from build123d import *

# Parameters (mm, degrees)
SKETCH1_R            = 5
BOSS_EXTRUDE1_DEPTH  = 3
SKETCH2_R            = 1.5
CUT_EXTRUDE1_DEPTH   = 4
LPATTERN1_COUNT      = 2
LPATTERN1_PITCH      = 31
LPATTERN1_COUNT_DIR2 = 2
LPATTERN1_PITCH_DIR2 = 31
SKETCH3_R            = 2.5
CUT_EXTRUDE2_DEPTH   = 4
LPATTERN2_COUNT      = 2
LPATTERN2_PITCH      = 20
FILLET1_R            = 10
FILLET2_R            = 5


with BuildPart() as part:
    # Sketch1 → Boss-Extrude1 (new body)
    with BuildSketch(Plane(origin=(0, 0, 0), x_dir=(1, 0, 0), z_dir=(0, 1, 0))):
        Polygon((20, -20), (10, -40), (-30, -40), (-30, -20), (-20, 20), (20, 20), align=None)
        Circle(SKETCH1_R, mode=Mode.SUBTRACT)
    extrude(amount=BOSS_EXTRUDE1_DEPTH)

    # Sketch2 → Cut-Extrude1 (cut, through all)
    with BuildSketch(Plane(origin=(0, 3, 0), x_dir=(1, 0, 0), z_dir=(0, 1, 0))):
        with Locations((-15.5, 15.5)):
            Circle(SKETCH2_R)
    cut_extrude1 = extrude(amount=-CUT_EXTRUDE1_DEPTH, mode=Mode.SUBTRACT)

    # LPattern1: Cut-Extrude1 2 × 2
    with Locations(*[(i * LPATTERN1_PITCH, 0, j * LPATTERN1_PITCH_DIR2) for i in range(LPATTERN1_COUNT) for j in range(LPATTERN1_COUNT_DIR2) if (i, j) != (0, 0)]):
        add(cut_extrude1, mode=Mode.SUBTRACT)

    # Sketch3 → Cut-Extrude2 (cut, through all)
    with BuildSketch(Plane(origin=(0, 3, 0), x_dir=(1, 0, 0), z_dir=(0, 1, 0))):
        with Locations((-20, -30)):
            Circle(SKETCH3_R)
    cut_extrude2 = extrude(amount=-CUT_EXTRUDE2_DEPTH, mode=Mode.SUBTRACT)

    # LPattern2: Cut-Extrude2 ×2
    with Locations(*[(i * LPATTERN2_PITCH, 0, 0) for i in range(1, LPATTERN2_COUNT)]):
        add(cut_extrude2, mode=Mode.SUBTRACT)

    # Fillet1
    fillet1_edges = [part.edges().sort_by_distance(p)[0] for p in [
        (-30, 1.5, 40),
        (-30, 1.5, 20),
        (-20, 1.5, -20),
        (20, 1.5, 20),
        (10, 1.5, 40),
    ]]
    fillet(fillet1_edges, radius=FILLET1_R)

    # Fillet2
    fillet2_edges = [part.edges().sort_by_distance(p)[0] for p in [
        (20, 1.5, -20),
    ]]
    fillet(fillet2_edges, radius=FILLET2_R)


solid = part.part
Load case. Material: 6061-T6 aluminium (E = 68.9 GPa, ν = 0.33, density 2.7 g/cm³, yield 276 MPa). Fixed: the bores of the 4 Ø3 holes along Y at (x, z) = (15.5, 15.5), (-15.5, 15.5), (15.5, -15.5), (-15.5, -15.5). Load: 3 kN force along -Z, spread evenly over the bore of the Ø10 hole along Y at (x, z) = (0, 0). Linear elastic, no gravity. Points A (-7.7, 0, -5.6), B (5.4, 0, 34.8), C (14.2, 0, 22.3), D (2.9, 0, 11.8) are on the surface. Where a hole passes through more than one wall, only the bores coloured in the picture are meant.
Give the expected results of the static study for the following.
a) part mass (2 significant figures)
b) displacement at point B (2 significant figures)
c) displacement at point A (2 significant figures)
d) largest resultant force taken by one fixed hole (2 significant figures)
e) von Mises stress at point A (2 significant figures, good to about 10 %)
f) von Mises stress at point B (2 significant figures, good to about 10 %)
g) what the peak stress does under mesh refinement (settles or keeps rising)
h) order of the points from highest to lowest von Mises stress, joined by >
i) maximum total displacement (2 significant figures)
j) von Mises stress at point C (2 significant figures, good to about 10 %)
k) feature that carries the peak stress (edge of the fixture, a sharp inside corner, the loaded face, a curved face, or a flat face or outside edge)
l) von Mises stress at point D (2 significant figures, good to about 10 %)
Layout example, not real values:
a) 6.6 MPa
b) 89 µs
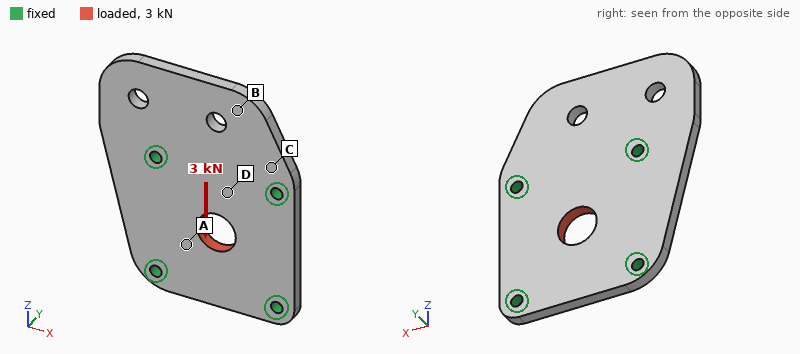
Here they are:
a) 20 g
b) 2.6 µm
c) 5.4 µm
d) 870 N
e) 24 MPa
f) 5.2 MPa
g) keeps rising
h) A > D > C > B
i) 9.7 µm
j) 11 MPa
k) edge of the fixture
l) 18 MPa
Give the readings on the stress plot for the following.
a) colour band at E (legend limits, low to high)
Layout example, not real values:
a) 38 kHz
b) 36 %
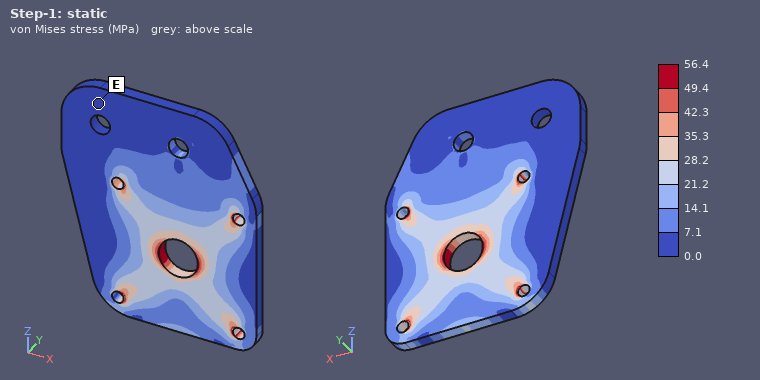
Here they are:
a) 0.0 to 7.1 MPa
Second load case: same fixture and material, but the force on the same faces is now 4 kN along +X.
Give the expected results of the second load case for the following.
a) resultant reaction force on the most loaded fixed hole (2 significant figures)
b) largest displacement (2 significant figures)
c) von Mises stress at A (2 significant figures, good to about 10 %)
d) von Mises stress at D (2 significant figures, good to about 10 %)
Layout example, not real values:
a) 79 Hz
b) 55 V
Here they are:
a) 1.2 kN
b) 13 µm
c) 33 MPa
d) 23 MPa
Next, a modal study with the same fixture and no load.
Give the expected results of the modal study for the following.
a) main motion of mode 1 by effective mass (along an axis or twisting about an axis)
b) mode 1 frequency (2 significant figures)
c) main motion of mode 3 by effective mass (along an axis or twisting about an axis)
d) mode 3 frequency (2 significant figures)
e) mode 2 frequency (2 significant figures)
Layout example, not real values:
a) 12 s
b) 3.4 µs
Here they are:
a) along Y
b) 4000 Hz
c) along Y
d) 11 kHz
e) 6500 Hz
